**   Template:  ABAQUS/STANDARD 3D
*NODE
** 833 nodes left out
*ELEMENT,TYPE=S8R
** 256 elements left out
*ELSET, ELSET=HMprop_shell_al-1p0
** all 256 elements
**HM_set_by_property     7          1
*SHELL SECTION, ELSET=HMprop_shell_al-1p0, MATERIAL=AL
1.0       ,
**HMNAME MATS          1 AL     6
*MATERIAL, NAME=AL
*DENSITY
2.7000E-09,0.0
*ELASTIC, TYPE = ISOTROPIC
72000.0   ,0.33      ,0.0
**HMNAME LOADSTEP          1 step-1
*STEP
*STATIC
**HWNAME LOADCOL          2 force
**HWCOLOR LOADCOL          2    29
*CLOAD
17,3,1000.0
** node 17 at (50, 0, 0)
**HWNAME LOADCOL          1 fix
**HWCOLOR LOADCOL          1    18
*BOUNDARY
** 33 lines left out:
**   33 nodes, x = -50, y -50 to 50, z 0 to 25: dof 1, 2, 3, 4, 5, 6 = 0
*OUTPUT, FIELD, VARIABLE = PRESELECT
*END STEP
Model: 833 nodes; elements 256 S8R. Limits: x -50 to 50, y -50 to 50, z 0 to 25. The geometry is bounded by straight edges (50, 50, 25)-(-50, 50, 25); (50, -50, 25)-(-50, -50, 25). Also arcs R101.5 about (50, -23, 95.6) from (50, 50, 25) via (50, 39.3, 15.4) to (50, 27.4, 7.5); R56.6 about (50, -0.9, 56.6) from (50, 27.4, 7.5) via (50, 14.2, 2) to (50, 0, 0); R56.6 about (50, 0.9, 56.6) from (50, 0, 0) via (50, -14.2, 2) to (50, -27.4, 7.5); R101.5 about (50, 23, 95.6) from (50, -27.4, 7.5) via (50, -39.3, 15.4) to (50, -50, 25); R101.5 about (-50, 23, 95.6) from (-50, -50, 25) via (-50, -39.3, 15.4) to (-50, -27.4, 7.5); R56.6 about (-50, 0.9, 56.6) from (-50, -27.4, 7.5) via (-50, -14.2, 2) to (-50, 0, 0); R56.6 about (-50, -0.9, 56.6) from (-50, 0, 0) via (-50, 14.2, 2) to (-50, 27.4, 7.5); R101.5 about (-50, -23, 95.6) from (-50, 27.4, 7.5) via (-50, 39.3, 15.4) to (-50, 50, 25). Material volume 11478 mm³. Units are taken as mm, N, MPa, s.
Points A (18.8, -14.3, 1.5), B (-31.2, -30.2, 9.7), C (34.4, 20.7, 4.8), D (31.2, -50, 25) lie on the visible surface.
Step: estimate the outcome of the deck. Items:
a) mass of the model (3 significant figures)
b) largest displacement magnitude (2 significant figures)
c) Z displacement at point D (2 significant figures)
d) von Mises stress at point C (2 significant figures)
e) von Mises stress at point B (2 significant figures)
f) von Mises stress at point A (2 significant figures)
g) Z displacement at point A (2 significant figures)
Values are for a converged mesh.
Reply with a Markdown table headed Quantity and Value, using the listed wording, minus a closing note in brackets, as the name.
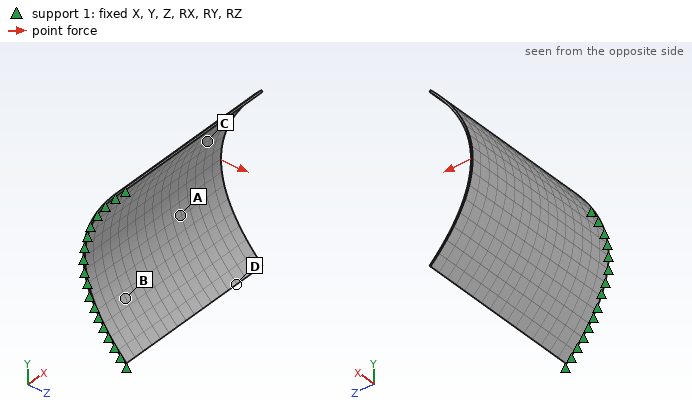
| Quantity | Value |
|---|---|
| mass of the model | 0.0310 kg |
| largest displacement magnitude | 8.5 mm |
| Z displacement at point D | -5.2 mm |
| von Mises stress at point C | 290 MPa |
| von Mises stress at point B | 150 MPa |
| von Mises stress at point A | 260 MPa |
| Z displacement at point A | 0.93 mm |
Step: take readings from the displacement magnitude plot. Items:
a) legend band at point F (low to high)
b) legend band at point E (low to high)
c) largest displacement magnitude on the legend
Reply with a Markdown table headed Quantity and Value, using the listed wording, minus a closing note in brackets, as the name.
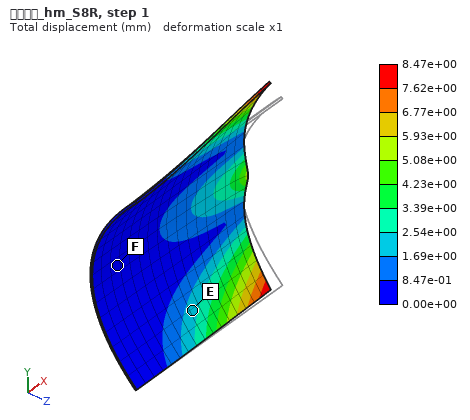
| Quantity | Value |
|---|---|
| legend band at point F | 0.00e+00 to 8.47e-01 mm |
| legend band at point E | 1.69e+00 to 2.54e+00 mm |
| largest displacement magnitude on the legend | 8.47e+00 mm |
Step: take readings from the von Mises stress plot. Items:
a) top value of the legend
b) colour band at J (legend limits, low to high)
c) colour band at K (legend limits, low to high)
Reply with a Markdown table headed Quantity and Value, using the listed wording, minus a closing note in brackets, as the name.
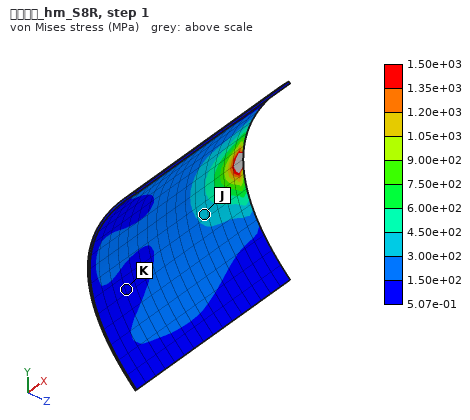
| Quantity | Value |
|---|---|
| top value of the legend | 1.50e+03 MPa |
| colour band at J | 3.00e+02 to 4.50e+02 MPa |
| colour band at K | 5.07e-01 to 1.50e+02 MPa |
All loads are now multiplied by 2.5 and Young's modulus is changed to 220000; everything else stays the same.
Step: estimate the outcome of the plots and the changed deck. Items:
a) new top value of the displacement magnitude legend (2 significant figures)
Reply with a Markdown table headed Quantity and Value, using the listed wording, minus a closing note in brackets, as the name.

| Quantity | Value |
|---|---|
| new top value of the displacement magnitude legend | 6.9 mm |
